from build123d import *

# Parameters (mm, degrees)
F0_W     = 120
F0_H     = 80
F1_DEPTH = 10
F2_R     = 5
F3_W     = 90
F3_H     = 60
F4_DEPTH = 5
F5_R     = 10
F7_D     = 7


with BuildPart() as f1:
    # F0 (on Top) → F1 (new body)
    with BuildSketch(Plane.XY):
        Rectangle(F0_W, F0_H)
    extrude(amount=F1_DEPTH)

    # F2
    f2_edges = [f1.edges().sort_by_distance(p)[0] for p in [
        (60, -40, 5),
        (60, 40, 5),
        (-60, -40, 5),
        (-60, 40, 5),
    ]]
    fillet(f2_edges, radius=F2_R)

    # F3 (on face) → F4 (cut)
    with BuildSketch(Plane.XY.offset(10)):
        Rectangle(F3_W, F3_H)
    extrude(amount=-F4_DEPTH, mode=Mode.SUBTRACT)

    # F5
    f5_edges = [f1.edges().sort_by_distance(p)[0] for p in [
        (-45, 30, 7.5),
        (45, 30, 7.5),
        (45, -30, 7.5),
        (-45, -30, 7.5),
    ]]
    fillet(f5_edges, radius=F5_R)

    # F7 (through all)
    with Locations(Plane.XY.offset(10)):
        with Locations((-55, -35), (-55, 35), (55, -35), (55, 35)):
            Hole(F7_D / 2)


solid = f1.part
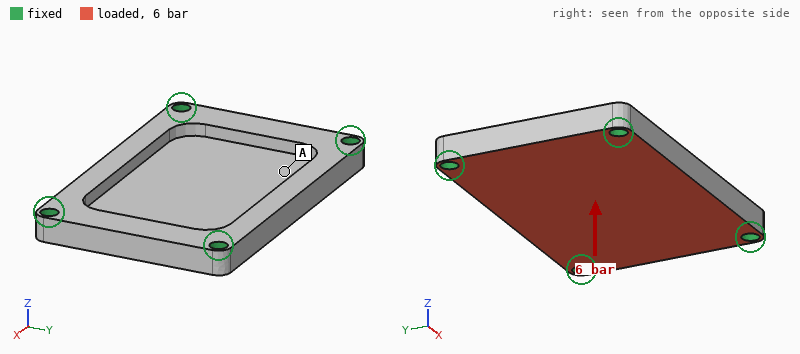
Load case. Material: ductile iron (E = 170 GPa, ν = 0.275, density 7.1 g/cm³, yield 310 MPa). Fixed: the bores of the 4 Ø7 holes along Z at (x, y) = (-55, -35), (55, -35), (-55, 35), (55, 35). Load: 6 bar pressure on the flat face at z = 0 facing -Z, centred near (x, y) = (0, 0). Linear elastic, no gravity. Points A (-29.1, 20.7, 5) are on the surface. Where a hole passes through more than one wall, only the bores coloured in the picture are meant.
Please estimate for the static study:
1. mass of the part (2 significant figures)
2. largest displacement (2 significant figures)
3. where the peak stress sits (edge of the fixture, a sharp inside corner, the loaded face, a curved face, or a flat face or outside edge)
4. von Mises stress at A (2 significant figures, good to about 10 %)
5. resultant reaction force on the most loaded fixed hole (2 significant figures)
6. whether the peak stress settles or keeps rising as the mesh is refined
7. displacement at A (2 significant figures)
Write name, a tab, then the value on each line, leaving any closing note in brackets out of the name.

mass of the part	480 g
largest displacement	56 µm
where the peak stress sits	edge of the fixture
von Mises stress at A	12 MPa
resultant reaction force on the most loaded fixed hole	1.7 kN
whether the peak stress settles or keeps rising as the mesh is refined	keeps rising
displacement at A	26 µm
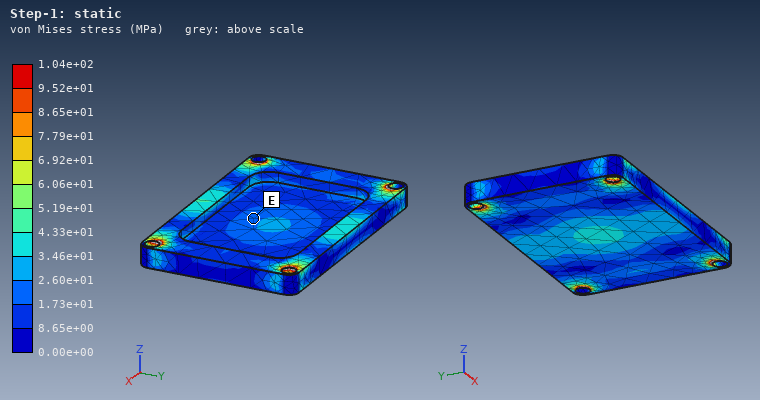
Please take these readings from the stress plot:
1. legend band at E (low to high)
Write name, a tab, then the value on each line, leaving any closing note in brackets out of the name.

legend band at E	1.73e+01 to 2.60e+01 MPa
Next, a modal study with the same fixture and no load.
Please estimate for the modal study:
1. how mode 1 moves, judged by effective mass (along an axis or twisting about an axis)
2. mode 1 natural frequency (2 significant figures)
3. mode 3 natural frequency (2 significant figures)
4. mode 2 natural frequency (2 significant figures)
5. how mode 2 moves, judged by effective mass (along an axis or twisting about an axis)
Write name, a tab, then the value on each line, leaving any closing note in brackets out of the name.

how mode 1 moves, judged by effective mass	along Z
mode 1 natural frequency	3200 Hz
mode 3 natural frequency	6600 Hz
mode 2 natural frequency	4500 Hz
how mode 2 moves, judged by effective mass	twisting about X
